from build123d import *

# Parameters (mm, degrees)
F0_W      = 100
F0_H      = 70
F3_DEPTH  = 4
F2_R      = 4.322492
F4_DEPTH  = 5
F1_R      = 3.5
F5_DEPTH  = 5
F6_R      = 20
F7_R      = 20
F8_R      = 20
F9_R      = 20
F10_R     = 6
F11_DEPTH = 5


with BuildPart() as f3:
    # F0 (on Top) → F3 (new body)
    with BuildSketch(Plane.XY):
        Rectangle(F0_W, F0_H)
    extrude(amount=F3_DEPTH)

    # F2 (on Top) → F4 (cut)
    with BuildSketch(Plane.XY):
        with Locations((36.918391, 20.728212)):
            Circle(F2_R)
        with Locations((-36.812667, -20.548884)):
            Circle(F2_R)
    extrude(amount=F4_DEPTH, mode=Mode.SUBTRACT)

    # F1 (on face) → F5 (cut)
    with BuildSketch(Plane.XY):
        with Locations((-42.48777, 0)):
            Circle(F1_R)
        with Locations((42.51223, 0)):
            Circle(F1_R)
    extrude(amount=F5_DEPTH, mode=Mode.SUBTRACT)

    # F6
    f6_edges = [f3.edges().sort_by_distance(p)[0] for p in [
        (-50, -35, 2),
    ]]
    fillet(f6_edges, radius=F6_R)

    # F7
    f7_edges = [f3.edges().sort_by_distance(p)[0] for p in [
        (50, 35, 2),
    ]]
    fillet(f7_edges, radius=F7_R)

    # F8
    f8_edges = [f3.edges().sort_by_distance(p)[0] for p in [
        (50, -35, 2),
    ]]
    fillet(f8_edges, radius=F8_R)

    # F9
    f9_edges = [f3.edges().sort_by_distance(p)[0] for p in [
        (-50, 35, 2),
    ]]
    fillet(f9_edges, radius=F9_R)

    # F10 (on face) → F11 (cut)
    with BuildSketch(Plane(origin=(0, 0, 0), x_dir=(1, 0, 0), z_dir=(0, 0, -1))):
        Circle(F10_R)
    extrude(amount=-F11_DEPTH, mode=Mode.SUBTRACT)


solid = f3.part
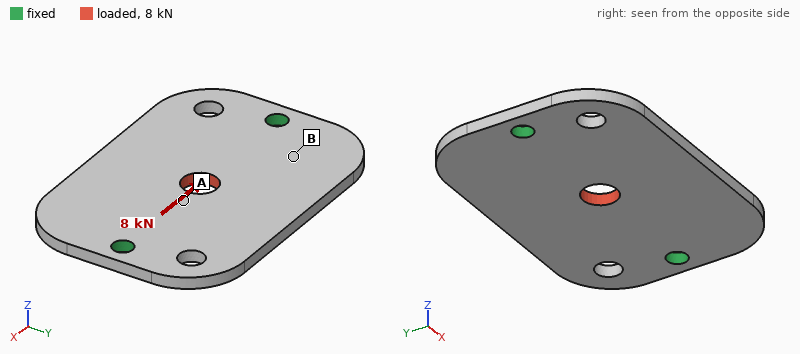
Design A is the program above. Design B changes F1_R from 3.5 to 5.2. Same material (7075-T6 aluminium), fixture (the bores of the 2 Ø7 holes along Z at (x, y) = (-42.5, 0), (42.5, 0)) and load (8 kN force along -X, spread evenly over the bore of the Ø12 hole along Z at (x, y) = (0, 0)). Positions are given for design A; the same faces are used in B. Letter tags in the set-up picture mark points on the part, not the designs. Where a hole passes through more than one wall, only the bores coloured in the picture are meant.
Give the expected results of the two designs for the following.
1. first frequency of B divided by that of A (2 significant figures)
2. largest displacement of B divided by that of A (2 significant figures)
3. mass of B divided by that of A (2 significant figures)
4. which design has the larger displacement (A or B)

1.1
0.90
0.99
A
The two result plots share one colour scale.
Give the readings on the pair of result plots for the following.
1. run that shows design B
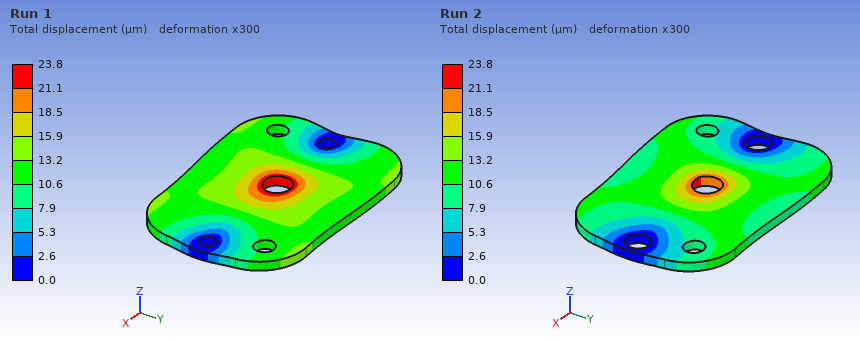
Run 2
